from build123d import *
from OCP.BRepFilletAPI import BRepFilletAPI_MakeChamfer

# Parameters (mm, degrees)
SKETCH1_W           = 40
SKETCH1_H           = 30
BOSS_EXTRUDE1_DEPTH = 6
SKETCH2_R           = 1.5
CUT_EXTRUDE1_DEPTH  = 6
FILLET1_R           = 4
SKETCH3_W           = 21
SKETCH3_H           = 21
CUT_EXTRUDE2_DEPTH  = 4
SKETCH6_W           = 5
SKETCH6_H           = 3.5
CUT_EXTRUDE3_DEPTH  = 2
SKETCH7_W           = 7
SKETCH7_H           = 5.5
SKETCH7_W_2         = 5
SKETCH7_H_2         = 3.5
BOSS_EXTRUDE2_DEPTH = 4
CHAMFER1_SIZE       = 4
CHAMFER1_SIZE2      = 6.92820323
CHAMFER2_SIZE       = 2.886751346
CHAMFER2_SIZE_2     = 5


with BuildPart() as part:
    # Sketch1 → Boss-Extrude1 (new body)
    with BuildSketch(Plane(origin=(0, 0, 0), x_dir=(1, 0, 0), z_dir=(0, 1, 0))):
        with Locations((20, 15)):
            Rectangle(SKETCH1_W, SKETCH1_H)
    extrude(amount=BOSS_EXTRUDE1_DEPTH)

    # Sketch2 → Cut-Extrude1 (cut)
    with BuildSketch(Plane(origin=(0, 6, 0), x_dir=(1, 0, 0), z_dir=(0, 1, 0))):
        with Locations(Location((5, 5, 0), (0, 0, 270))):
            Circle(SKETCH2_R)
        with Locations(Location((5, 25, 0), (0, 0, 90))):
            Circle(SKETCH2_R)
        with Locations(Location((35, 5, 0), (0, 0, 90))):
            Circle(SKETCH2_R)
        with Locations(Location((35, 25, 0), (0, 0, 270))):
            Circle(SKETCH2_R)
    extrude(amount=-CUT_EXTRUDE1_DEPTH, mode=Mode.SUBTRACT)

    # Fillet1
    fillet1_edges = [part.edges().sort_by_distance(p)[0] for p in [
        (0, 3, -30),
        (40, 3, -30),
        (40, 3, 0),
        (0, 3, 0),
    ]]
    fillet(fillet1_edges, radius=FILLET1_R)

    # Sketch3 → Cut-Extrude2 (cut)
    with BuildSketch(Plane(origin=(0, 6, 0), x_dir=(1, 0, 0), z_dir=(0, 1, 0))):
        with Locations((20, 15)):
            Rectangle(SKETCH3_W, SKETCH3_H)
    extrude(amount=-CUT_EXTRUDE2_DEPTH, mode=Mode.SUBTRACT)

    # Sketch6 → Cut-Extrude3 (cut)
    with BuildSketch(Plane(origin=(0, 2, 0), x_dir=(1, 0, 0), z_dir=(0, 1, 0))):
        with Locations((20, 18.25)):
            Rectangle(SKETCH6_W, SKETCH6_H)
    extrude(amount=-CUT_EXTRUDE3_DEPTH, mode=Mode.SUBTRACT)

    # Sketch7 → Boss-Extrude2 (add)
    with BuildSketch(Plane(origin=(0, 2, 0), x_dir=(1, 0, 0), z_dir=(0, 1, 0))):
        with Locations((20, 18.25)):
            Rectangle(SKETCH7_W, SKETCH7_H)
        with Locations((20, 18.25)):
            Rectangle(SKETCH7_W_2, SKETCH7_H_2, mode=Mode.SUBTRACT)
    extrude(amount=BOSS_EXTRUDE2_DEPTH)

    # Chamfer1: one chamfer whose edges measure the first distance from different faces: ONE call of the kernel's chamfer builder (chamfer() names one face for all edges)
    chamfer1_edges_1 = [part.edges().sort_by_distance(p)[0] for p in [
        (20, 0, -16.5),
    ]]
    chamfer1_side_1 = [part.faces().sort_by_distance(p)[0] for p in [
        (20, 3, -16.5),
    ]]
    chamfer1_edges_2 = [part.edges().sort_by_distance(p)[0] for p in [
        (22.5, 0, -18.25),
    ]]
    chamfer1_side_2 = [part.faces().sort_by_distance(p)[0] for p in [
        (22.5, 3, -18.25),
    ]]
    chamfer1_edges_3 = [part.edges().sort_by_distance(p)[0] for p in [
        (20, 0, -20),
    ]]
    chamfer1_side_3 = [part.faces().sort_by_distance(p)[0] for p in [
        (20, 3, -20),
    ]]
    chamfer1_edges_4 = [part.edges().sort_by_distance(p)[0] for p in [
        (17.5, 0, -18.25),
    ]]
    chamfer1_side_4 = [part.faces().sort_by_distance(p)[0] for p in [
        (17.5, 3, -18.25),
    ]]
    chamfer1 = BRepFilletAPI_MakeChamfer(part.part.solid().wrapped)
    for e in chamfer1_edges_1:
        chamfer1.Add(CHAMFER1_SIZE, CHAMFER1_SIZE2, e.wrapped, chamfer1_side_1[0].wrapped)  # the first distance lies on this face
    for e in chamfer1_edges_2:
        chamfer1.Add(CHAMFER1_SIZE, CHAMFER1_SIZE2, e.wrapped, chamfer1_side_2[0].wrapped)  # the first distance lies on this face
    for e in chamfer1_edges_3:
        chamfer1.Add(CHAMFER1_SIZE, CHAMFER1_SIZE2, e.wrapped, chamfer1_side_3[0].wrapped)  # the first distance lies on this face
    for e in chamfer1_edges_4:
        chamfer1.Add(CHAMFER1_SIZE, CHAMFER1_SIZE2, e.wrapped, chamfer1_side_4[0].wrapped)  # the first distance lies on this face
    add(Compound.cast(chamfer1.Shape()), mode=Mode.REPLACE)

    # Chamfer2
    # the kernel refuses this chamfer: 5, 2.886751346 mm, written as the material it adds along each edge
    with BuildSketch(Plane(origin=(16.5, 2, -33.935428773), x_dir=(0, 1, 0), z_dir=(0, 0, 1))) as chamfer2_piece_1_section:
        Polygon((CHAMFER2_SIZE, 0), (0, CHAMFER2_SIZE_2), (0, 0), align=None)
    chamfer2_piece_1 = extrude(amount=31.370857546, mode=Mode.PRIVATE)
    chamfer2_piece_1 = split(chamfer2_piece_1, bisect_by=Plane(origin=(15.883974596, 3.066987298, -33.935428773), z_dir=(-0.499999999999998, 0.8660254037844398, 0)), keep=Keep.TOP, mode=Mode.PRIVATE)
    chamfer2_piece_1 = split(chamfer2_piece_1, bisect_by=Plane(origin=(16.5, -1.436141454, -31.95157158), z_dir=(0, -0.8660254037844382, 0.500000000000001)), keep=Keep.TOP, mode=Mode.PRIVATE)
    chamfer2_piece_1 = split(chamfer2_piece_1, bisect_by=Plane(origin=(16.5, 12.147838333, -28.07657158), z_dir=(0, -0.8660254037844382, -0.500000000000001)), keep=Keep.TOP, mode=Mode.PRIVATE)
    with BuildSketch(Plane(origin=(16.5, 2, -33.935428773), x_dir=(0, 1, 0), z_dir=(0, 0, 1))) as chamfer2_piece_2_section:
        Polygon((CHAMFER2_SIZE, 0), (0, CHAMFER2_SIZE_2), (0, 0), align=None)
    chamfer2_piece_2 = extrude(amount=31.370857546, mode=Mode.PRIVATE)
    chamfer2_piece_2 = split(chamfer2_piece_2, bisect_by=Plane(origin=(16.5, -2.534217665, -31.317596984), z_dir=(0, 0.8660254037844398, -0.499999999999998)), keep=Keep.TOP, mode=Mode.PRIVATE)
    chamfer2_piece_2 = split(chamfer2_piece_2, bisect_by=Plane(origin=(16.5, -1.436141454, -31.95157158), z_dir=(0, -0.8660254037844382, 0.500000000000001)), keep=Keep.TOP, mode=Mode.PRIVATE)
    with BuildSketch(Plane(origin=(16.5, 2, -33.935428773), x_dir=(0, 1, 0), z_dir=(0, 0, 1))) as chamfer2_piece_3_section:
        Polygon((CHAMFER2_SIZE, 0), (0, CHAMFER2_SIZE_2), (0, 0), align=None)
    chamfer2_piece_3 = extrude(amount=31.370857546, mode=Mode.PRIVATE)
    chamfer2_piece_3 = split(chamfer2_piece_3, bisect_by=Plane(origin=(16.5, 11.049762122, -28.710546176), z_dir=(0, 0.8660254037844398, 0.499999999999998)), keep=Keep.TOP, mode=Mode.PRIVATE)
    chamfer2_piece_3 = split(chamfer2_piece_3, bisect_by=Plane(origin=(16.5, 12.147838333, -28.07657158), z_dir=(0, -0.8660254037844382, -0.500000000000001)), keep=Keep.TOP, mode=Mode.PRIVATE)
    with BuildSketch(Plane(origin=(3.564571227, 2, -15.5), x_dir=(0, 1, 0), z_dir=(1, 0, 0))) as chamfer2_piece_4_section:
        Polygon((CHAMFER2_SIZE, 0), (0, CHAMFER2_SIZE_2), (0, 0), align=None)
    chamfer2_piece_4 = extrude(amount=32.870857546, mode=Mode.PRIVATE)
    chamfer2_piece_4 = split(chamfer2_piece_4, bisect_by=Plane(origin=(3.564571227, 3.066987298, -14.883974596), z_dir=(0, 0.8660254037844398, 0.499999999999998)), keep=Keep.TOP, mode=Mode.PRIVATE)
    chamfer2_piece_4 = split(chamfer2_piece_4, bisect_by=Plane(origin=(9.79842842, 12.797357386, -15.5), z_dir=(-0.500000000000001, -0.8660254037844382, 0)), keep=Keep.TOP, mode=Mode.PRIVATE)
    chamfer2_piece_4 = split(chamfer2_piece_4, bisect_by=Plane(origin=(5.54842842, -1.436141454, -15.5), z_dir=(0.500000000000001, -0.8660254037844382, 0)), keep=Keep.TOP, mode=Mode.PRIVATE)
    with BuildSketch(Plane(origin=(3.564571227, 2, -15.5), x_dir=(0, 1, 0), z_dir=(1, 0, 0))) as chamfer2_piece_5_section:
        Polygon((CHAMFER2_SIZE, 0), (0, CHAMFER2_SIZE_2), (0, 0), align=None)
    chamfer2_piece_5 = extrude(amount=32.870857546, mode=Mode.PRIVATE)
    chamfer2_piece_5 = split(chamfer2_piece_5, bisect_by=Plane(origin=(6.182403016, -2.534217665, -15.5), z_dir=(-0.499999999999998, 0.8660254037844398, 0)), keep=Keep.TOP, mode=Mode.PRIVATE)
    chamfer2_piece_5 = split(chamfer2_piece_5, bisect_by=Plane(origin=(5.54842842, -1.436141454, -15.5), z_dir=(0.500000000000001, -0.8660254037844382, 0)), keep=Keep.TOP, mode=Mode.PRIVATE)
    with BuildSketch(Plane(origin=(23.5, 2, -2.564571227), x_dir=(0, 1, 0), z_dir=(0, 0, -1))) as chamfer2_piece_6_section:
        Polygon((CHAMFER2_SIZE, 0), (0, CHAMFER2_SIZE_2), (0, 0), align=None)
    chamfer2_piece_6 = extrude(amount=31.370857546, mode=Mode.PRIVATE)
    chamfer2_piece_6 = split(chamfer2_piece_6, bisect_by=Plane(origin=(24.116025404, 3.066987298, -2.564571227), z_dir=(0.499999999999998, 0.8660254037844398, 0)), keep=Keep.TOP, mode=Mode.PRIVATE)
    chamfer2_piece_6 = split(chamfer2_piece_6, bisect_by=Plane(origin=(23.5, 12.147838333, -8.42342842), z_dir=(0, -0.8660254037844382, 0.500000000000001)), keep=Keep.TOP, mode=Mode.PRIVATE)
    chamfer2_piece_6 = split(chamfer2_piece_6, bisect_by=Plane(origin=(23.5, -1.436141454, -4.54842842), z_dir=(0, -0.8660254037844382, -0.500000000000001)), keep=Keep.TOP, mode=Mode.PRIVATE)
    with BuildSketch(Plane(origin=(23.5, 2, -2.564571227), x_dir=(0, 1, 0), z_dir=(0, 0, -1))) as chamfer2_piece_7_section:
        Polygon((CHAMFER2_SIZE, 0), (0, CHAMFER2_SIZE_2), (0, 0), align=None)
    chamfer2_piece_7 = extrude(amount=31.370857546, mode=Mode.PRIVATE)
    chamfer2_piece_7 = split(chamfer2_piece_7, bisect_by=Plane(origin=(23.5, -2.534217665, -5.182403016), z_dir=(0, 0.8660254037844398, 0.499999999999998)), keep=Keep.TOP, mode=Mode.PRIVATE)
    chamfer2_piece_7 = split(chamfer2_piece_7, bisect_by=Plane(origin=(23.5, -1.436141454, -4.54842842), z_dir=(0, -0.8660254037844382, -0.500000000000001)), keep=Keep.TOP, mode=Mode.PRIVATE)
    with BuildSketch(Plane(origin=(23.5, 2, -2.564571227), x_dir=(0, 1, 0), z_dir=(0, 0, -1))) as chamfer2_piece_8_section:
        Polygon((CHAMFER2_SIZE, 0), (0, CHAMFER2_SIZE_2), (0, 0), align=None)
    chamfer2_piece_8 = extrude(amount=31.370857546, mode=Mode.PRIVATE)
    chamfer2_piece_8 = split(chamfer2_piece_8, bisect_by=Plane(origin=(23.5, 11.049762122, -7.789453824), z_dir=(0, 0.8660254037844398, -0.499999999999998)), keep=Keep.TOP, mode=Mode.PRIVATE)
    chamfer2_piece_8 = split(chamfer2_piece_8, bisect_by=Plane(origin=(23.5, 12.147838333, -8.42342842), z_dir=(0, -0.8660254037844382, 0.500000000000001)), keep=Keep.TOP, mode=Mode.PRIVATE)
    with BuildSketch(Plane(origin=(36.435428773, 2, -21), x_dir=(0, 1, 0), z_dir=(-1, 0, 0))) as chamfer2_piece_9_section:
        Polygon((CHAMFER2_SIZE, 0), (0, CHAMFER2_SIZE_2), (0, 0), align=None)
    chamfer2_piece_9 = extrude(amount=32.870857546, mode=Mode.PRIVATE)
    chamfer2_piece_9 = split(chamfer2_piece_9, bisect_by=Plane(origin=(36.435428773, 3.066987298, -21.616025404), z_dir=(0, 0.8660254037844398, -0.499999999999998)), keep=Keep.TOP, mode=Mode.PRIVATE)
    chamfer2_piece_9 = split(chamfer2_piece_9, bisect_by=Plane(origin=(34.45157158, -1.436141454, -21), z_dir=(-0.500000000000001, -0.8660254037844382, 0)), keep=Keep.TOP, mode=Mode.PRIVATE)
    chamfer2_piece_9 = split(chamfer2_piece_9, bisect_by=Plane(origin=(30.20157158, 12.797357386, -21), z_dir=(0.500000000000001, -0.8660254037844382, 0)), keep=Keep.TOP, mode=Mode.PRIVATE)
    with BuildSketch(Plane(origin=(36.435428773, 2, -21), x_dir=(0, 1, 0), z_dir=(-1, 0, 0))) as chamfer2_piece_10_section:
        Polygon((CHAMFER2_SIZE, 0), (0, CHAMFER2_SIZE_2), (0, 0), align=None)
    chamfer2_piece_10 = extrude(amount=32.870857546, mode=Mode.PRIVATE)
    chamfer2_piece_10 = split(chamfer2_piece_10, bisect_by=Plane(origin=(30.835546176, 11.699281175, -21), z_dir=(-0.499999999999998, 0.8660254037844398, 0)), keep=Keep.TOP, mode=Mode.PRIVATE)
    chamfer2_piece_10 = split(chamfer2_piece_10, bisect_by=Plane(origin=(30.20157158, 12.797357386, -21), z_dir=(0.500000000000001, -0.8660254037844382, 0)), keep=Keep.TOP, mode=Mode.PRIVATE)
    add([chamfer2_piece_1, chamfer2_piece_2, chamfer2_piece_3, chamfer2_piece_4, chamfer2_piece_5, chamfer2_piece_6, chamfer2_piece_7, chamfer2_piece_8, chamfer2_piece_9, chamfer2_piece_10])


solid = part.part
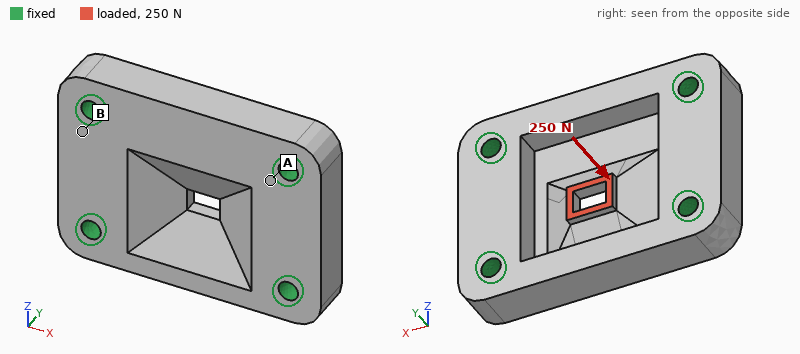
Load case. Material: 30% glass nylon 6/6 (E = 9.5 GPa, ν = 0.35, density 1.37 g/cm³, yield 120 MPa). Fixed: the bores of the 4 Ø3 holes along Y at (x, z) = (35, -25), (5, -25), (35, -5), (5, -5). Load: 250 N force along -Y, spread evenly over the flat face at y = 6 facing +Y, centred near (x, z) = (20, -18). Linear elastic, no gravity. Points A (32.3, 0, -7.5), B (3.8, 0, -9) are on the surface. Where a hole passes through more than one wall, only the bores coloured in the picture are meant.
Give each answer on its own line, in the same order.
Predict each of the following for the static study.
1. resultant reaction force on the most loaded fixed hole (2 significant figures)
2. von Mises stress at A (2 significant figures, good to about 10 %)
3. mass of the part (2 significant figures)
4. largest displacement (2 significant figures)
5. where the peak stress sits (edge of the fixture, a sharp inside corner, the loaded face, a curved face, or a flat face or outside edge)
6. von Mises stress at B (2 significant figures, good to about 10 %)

110 N
8.9 MPa
6.9 g
67 µm
the loaded face
4.2 MPa
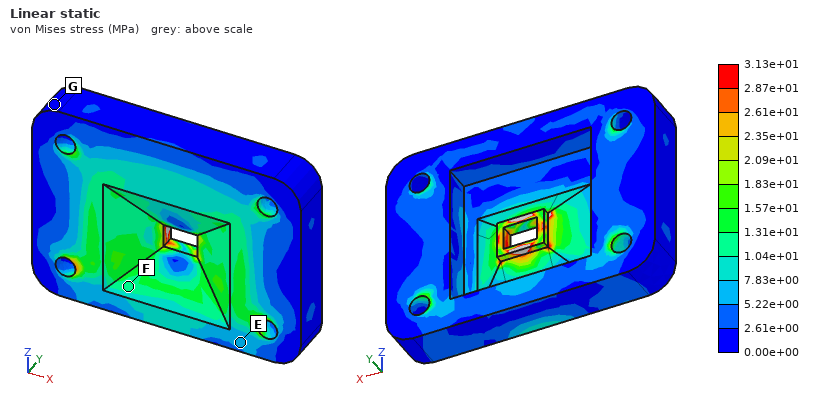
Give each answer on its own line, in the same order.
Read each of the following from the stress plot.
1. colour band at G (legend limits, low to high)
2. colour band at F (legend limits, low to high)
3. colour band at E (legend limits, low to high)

0.00e+00 to 2.61e+00 MPa
1.04e+01 to 1.31e+01 MPa
5.22e+00 to 7.83e+00 MPa
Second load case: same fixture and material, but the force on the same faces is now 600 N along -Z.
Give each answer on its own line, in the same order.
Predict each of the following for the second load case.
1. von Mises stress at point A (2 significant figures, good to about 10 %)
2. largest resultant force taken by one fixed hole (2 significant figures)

17 MPa
190 N
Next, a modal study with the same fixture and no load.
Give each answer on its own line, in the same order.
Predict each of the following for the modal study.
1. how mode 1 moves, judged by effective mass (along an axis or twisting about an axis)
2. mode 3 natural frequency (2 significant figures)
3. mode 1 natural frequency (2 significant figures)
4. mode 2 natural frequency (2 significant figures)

along Y
18 kHz
14 kHz
16 kHz
